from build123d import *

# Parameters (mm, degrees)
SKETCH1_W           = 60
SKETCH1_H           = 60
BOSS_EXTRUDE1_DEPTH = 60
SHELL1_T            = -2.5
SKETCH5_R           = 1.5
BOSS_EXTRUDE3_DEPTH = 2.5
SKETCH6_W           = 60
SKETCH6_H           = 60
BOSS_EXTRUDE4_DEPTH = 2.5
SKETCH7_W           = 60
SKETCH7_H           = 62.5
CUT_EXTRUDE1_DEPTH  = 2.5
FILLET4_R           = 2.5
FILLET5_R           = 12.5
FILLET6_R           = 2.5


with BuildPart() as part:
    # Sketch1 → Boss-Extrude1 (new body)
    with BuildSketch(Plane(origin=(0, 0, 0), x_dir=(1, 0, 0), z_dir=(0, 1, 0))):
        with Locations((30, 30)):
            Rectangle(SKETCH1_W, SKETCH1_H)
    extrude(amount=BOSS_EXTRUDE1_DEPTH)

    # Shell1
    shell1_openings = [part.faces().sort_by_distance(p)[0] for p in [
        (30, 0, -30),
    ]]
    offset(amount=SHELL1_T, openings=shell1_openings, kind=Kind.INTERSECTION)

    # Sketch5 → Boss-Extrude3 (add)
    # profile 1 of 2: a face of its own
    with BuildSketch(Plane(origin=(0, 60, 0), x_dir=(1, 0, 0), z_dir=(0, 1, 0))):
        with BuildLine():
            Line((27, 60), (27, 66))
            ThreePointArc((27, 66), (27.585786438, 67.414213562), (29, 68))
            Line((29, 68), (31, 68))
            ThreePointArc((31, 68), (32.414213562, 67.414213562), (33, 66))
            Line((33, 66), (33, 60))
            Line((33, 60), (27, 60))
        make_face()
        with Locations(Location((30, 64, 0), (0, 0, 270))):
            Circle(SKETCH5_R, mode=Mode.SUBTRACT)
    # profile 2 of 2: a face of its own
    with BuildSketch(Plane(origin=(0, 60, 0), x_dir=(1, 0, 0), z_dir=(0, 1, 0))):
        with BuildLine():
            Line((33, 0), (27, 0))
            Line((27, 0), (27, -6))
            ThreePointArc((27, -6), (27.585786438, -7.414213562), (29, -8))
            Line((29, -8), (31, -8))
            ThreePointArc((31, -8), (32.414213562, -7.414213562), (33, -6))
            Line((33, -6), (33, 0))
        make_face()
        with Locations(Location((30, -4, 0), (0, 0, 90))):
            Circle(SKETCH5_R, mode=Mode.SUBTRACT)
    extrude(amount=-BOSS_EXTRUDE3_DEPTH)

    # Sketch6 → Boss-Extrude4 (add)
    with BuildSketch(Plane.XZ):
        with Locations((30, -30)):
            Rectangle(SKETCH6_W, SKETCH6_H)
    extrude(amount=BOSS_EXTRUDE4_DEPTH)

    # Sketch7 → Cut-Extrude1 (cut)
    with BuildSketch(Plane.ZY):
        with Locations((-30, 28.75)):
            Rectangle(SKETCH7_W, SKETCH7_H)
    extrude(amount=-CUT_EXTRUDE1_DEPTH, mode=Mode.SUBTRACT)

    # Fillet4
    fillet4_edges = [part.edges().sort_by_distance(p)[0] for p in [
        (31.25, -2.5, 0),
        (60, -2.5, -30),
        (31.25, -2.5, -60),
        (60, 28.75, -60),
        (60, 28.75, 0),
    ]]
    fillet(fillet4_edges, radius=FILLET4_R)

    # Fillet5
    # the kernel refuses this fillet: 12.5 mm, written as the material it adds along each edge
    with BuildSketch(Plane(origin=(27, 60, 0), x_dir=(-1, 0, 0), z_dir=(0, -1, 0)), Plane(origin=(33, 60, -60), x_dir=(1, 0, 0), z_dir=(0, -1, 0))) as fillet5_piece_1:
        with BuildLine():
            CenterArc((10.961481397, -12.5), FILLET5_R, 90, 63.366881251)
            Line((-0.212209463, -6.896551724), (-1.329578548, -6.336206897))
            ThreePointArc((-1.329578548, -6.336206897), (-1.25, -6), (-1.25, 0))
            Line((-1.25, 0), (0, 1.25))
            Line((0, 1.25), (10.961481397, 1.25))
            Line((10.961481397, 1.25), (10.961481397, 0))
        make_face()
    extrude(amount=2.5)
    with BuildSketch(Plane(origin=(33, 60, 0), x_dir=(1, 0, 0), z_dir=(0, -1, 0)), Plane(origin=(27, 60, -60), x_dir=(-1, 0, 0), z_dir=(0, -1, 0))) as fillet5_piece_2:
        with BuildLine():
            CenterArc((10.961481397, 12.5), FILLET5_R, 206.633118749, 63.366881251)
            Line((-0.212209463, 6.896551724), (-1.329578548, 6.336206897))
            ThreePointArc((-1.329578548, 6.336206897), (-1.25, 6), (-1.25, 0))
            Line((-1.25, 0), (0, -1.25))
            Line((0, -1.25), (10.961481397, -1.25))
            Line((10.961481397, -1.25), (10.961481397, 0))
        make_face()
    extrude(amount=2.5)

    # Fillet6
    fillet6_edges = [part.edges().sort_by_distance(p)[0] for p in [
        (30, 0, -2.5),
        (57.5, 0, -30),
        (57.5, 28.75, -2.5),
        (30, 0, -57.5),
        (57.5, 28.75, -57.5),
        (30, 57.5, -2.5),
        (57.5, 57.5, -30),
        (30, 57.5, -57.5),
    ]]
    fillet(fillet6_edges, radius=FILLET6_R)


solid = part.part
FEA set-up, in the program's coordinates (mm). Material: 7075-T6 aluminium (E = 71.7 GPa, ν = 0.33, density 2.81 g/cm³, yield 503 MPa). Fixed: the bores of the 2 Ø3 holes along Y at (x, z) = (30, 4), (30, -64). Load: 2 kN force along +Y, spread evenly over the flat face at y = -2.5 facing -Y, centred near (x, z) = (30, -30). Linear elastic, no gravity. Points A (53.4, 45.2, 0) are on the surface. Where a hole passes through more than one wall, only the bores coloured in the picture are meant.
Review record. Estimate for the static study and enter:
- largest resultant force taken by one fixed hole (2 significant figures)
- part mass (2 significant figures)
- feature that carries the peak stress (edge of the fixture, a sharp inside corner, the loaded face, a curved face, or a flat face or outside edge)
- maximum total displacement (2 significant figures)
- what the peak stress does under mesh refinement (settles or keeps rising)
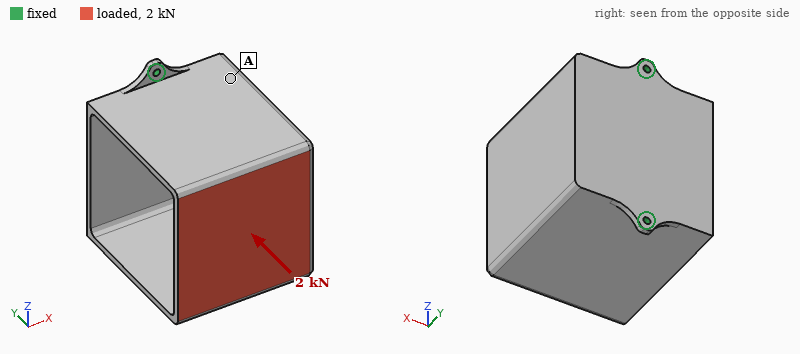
1.0 kN
120 g
edge of the fixture
0.43 mm
keeps rising
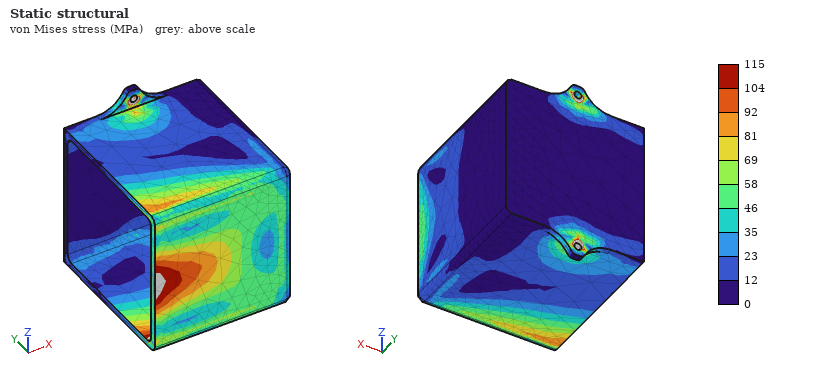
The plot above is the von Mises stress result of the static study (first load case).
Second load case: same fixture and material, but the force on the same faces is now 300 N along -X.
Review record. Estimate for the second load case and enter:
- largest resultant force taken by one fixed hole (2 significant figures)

150 N
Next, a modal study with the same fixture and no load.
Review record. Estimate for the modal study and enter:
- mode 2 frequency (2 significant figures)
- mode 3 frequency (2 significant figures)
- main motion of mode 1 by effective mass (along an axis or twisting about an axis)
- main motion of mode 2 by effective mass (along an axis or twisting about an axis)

650 Hz
2300 Hz
along X
along Z
